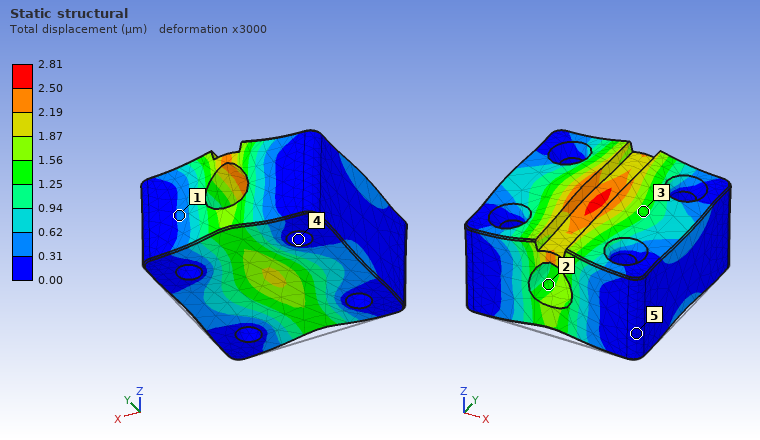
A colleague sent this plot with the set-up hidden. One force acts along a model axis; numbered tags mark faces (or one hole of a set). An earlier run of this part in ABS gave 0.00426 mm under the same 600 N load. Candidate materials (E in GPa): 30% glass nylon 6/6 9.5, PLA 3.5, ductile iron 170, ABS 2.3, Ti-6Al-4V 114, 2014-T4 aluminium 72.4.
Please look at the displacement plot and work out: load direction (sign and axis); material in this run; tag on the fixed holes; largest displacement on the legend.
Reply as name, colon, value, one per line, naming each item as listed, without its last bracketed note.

load direction: +Z
material in this run: PLA
tag on the fixed holes: 4
largest displacement on the legend: 2.81 µm
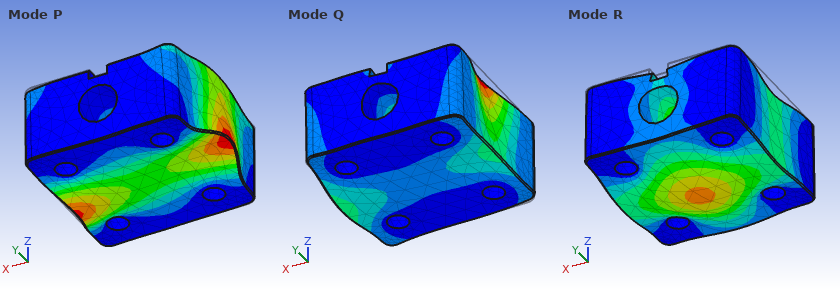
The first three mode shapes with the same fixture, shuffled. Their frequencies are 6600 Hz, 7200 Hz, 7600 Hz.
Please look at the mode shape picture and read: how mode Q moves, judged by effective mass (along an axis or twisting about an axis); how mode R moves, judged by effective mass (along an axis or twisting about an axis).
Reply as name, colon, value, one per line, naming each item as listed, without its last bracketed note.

how mode Q moves, judged by effective mass: along X
how mode R moves, judged by effective mass: along Z
